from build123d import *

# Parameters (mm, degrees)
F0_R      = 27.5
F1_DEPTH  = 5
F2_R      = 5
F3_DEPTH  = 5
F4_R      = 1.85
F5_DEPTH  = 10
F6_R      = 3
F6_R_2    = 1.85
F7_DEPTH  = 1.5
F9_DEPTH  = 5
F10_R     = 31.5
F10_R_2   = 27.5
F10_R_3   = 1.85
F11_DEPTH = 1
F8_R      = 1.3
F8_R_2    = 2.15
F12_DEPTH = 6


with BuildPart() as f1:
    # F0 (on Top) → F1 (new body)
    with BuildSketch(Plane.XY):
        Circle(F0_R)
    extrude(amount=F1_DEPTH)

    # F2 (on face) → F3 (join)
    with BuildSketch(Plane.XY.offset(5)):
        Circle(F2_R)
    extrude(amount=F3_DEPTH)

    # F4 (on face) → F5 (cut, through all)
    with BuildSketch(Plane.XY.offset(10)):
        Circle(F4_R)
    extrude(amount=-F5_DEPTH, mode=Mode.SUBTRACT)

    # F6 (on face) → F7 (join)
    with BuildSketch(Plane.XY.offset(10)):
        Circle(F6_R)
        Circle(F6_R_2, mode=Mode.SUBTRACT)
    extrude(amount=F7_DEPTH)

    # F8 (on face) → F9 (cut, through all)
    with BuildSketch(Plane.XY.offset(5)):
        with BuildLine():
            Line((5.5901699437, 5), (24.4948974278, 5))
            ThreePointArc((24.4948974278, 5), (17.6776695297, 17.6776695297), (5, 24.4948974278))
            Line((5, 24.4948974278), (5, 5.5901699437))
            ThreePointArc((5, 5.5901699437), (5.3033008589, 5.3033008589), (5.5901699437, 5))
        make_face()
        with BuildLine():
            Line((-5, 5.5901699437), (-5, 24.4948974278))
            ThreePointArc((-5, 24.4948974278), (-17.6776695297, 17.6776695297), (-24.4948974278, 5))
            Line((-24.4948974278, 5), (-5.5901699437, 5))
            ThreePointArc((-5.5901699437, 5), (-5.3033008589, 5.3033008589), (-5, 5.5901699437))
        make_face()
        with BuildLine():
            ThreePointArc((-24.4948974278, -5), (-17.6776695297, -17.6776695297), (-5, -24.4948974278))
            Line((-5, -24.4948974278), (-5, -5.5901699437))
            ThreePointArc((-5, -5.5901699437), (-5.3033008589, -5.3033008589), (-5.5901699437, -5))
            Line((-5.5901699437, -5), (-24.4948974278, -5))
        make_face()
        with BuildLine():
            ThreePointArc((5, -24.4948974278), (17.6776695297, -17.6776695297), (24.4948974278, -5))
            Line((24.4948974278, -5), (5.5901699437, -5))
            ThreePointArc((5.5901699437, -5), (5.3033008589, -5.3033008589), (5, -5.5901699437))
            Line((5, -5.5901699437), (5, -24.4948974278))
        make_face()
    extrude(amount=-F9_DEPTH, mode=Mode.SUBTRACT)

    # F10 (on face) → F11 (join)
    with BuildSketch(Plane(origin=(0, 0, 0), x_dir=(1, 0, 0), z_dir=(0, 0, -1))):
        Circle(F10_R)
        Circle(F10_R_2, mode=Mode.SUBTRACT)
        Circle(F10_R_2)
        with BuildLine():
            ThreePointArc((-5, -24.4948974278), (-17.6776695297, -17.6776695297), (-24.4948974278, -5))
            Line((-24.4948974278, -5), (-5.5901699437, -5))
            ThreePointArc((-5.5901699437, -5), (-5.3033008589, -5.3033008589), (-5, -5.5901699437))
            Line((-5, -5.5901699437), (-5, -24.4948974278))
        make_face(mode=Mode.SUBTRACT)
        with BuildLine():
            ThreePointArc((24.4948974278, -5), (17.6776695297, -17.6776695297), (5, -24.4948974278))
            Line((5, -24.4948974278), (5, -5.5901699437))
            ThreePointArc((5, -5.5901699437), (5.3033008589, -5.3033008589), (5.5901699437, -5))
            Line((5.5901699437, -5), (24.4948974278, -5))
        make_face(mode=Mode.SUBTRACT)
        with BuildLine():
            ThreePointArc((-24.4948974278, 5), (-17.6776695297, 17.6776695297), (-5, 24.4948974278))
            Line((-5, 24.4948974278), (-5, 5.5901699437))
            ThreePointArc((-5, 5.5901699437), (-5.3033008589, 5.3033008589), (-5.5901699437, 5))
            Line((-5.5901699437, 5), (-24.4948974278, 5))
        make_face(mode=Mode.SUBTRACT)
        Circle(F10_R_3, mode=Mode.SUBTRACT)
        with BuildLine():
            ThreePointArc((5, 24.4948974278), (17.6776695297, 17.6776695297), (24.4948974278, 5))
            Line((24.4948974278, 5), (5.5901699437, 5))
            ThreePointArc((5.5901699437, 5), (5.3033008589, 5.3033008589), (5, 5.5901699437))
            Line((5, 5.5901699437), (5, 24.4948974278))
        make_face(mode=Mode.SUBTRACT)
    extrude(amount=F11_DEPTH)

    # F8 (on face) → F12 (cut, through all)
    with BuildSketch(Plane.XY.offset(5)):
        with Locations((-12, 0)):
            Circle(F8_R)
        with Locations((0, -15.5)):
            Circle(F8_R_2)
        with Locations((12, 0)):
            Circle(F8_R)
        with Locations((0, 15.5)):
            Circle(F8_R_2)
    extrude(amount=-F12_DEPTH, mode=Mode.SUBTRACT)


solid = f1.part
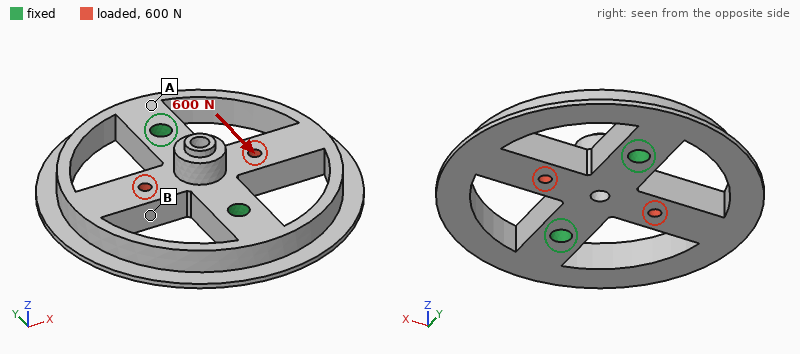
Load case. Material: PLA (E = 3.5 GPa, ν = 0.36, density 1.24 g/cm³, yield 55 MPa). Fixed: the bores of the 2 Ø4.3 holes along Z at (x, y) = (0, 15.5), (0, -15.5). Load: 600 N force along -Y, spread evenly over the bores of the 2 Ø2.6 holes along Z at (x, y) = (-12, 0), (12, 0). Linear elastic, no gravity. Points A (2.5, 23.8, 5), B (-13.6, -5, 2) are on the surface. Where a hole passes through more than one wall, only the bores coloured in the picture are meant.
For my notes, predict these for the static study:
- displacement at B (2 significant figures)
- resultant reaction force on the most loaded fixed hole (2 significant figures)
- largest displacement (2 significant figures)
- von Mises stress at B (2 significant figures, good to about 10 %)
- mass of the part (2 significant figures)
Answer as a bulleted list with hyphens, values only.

- 68 µm
- 300 N
- 78 µm
- 8.8 MPa
- 11 g
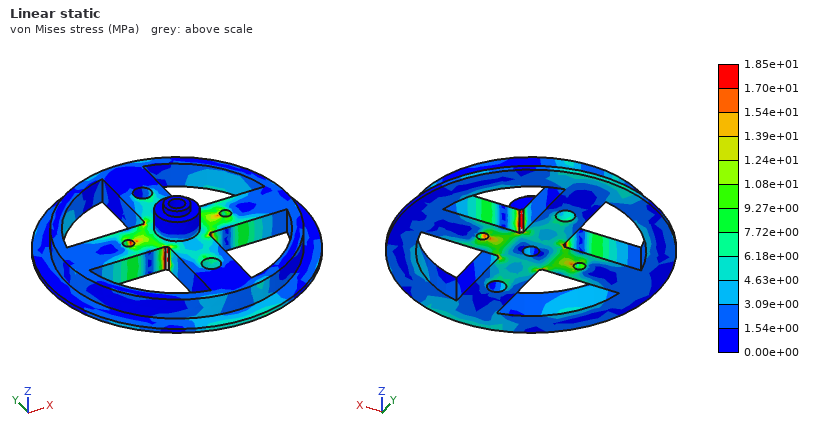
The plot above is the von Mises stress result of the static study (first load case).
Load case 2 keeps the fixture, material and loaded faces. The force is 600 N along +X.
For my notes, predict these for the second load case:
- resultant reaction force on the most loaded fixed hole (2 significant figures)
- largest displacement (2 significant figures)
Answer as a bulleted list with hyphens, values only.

- 300 N
- 78 µm
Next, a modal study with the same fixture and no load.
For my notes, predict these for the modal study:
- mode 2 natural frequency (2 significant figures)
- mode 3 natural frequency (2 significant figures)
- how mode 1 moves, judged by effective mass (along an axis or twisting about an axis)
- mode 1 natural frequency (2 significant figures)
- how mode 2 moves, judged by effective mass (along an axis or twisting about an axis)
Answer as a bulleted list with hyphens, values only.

- 1800 Hz
- 2900 Hz
- twisting about Y
- 1300 Hz
- along Z
